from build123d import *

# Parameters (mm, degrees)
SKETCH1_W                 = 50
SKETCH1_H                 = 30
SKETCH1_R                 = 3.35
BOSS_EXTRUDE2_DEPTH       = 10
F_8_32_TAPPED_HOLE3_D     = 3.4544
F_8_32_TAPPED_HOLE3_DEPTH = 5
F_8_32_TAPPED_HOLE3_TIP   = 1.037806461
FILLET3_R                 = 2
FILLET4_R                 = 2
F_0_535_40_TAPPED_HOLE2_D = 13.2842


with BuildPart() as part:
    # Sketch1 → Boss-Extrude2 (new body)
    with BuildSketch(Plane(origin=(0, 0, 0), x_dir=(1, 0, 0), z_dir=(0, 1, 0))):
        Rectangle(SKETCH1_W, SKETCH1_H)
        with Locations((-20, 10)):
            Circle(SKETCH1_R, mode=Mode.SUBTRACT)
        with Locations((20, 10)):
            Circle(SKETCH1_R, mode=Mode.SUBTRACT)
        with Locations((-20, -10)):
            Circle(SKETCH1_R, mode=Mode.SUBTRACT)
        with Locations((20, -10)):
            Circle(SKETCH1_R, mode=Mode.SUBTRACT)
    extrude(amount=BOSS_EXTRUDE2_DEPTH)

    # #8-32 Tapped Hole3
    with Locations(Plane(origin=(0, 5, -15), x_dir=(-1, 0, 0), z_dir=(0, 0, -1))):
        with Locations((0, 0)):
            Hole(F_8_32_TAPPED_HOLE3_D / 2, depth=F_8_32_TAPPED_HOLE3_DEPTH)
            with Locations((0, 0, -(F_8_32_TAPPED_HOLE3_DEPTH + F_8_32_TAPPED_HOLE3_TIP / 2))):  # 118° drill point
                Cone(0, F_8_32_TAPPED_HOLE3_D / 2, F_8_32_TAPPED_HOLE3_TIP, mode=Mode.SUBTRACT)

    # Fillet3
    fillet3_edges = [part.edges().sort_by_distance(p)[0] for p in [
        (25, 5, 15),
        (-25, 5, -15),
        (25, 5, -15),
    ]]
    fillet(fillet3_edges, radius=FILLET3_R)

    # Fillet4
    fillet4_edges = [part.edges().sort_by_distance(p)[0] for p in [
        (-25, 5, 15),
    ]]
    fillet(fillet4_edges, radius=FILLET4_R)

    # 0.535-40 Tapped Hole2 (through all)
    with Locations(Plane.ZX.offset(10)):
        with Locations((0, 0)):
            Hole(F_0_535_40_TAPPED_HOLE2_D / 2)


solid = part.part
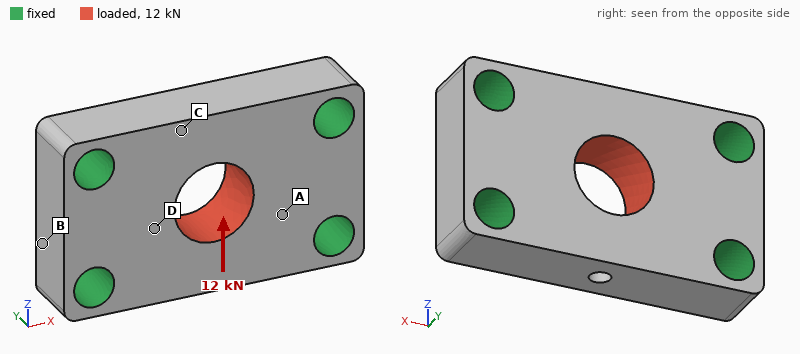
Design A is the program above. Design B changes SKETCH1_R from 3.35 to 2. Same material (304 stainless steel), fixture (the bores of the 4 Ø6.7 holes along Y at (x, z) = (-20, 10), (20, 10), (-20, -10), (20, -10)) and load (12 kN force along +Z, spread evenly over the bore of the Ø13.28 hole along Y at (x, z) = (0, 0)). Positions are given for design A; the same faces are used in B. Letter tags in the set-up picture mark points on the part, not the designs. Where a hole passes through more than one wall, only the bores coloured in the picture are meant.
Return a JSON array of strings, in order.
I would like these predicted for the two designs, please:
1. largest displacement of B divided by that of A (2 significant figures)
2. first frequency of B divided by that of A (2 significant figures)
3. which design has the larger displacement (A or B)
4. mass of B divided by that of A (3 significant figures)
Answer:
["1.1", "0.84", "B", "1.07"]
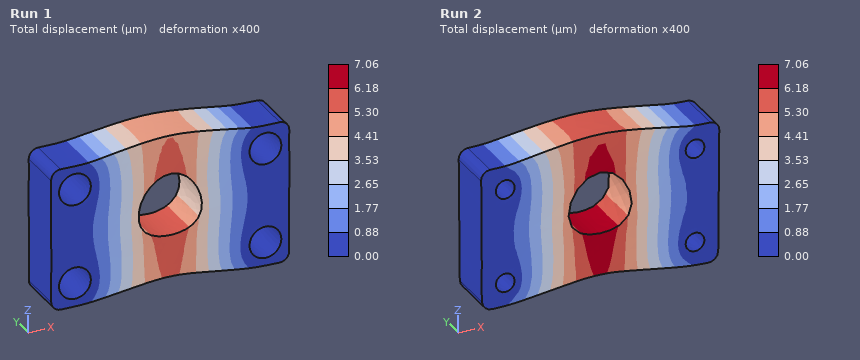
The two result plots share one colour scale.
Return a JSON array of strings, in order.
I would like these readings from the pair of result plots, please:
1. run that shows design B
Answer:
["Run 2"]
